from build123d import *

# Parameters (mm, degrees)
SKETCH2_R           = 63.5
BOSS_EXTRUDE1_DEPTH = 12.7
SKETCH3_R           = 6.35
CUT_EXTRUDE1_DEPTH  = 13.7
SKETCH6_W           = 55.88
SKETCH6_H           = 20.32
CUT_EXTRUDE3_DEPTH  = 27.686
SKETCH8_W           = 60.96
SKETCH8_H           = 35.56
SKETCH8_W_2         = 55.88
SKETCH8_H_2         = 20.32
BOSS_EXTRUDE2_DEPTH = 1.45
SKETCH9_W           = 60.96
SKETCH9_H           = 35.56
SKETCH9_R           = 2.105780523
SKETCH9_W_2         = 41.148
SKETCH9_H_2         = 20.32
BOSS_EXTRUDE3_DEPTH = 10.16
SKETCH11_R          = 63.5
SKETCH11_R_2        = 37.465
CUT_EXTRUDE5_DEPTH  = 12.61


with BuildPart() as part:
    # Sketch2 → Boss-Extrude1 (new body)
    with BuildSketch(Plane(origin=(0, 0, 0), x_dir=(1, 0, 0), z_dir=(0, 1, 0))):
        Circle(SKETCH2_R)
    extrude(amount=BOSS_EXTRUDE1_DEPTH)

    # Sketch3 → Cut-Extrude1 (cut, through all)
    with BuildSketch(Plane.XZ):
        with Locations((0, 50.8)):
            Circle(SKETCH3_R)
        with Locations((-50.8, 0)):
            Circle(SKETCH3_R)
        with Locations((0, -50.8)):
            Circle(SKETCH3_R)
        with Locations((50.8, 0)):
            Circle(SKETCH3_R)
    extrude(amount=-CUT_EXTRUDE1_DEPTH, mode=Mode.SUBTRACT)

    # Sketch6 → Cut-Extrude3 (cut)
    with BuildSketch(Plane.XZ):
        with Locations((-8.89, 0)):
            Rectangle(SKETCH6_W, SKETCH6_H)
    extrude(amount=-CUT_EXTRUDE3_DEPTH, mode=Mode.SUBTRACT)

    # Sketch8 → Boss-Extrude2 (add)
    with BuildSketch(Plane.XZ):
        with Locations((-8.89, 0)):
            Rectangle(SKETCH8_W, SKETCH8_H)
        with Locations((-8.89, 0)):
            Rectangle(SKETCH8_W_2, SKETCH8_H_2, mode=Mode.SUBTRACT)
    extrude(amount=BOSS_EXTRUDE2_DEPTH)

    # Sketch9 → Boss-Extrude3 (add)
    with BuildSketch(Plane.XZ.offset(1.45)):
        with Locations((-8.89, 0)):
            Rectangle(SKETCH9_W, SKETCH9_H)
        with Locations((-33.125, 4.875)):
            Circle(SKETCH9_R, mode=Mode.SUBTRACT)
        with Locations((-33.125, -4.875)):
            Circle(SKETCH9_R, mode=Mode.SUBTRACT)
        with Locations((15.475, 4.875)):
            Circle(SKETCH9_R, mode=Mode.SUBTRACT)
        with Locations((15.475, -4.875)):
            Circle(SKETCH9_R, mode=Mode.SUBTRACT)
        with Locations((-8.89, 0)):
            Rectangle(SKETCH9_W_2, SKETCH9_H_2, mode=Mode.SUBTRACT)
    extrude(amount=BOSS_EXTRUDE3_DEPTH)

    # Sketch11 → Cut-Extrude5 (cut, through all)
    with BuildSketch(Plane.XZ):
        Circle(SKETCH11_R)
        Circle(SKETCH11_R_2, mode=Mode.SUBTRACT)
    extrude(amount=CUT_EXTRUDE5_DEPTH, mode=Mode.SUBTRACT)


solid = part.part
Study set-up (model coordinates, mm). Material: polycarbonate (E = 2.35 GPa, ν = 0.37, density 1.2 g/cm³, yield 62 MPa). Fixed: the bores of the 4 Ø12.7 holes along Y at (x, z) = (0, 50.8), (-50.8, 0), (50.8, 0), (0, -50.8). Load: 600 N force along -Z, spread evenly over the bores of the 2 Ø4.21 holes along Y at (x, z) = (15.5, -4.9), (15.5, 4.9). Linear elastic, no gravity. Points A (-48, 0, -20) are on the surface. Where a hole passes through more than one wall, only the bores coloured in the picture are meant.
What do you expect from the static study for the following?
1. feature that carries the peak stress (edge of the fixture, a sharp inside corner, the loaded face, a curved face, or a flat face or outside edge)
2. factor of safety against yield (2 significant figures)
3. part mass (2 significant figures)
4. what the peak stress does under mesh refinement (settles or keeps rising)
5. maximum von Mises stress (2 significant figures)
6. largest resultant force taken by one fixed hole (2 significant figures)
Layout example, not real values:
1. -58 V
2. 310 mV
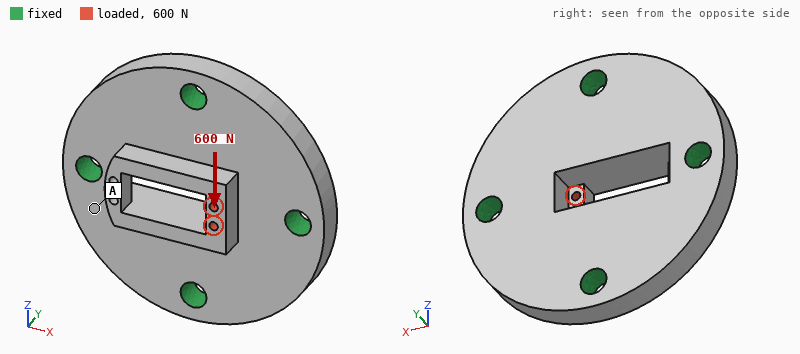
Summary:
1. the loaded face
2. 5.3
3. 180 g
4. settles
5. 12 MPa
6. 220 N
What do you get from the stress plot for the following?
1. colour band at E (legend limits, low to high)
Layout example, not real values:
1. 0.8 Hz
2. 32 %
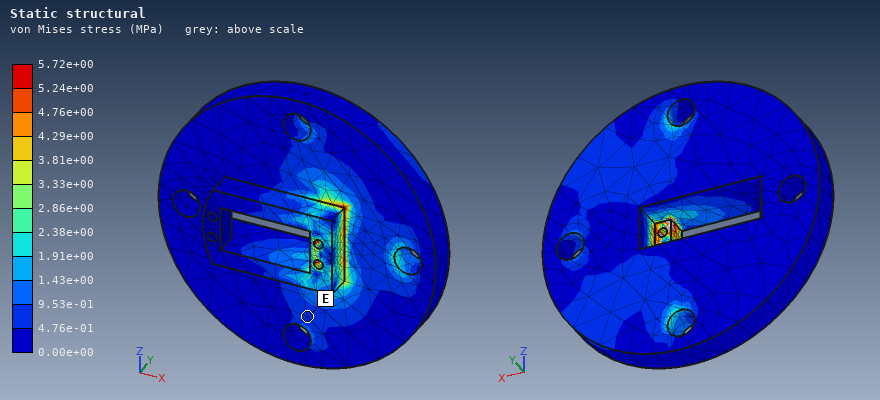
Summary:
1. 4.76e-01 to 9.53e-01 MPa
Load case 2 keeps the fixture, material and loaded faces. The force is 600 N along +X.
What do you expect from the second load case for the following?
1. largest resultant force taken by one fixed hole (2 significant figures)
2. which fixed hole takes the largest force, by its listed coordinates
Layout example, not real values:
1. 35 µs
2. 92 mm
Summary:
1. 290 N
2. (50.8, 0)
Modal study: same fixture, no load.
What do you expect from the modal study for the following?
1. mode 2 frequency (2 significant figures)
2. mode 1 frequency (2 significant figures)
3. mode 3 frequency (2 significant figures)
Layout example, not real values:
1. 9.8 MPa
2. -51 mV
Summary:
1. 2700 Hz
2. 2600 Hz
3. 2700 Hz
